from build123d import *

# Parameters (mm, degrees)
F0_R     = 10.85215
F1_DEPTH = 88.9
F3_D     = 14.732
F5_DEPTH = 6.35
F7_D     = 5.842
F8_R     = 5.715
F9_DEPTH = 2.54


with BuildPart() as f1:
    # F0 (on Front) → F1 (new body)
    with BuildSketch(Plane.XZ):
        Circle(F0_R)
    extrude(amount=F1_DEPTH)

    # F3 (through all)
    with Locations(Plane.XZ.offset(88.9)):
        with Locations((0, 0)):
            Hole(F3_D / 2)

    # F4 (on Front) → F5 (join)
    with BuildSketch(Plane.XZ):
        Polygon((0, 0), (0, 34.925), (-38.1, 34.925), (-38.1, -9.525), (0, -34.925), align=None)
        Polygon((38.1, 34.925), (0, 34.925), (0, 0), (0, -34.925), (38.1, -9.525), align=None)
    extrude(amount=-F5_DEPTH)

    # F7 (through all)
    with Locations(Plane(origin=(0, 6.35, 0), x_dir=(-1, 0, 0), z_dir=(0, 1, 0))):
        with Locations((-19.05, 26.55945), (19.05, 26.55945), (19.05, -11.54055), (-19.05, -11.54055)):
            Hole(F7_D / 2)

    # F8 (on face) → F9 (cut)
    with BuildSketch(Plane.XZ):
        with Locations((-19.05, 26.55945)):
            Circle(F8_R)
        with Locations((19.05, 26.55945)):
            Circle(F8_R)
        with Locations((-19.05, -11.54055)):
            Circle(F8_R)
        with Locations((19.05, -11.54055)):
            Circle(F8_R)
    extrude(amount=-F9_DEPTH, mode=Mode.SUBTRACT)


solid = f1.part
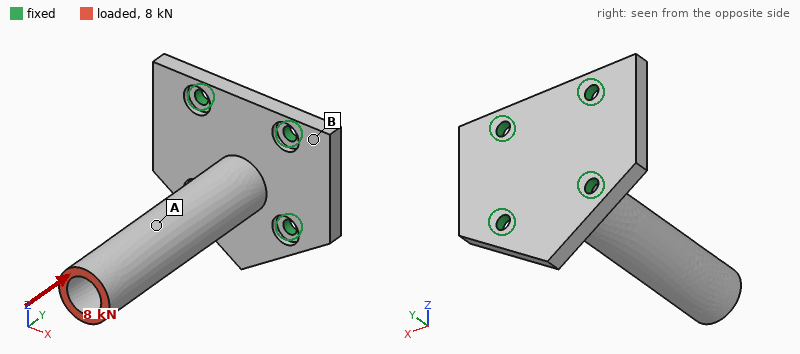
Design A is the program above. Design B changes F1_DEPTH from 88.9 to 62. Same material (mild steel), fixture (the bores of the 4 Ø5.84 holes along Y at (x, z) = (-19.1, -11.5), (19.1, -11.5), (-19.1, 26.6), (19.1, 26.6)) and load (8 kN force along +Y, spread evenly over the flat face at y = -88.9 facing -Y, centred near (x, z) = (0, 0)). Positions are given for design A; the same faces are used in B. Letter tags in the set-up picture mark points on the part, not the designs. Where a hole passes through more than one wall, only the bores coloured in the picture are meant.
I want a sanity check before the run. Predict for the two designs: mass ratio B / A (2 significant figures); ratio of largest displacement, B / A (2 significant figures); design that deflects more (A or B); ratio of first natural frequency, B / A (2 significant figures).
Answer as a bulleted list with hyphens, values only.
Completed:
- 0.95
- 0.75
- A
- 1.8
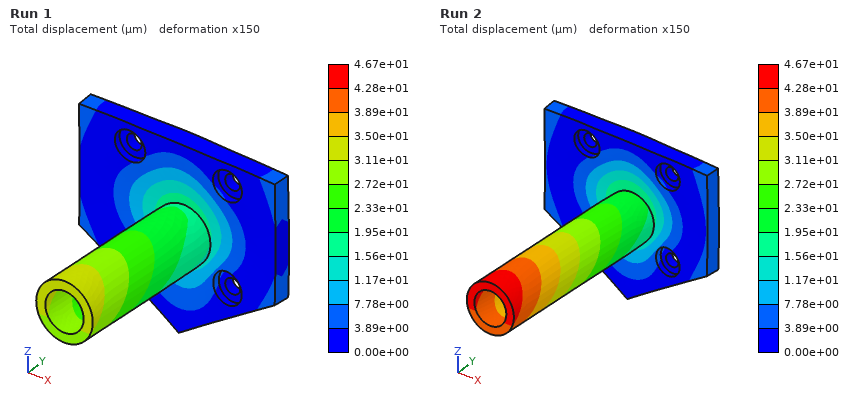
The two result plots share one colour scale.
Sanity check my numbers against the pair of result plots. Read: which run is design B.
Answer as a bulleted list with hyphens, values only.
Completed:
- Run 1
